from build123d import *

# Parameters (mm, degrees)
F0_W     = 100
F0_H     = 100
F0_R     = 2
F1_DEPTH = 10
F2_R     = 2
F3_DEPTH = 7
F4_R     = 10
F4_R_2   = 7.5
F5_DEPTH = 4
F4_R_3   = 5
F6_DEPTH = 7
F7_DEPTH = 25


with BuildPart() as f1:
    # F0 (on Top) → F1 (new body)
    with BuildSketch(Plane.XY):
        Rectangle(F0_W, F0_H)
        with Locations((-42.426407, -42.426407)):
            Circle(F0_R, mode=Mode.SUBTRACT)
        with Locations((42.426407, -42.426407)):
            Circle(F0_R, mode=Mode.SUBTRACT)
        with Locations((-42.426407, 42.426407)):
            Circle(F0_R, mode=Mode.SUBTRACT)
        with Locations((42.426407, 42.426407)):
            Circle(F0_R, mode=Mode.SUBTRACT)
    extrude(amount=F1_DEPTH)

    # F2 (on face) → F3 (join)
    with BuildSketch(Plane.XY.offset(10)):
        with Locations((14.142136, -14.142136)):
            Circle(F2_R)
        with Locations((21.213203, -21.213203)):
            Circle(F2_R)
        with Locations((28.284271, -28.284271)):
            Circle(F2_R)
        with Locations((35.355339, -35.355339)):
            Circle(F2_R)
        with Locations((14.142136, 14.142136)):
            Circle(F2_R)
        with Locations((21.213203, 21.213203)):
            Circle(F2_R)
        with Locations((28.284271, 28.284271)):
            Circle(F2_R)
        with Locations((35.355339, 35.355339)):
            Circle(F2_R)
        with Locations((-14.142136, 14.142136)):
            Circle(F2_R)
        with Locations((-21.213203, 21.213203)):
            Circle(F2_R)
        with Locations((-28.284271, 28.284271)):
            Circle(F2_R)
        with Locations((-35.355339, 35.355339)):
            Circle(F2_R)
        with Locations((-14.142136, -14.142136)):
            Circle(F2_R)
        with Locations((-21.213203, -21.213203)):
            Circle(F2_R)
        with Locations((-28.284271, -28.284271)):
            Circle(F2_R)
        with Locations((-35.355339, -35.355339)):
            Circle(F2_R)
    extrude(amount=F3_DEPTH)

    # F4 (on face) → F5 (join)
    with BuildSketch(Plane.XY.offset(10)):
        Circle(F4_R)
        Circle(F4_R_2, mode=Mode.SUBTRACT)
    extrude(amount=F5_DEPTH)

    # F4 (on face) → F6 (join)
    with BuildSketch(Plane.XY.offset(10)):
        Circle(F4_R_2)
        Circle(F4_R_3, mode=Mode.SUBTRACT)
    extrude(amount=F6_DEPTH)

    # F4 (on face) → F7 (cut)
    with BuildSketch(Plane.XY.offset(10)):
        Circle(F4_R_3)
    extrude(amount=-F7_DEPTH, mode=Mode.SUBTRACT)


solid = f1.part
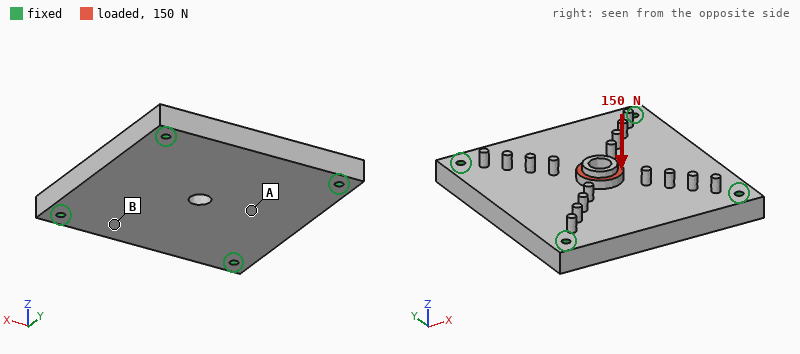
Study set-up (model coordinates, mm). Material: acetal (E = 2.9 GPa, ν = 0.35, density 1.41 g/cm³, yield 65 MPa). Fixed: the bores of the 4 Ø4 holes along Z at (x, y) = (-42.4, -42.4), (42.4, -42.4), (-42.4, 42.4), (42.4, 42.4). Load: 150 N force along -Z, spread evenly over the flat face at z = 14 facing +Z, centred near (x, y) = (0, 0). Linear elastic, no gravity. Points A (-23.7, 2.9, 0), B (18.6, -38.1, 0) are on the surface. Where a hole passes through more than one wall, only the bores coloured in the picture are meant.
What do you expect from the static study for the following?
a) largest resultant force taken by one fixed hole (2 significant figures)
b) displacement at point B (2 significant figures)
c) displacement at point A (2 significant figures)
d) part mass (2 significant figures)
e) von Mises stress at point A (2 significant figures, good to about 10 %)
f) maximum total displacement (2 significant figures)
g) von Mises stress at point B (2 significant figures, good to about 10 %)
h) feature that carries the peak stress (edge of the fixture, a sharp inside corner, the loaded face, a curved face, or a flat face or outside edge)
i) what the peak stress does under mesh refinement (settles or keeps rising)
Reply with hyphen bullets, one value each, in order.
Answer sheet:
- 38 N
- 23 µm
- 48 µm
- 140 g
- 0.90 MPa
- 68 µm
- 0.39 MPa
- edge of the fixture
- keeps rising
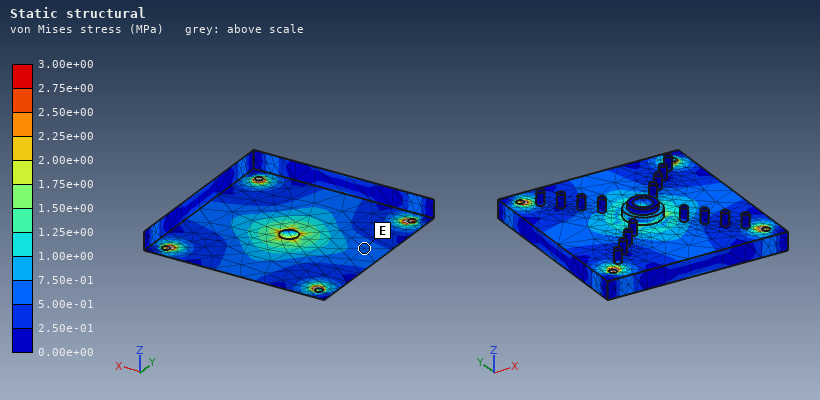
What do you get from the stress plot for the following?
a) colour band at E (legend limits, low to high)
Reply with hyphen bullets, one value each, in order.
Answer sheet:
- 5.00e-01 to 7.50e-01 MPa
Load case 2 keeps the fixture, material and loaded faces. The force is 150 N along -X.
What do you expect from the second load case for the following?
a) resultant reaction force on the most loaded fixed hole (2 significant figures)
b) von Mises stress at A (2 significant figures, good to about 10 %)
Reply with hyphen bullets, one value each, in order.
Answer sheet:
- 43 N
- 0.28 MPa
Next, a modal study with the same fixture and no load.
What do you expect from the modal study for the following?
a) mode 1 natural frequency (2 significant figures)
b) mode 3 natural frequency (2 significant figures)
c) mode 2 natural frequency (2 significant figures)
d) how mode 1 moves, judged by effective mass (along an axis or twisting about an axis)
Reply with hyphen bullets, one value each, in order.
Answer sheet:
- 1100 Hz
- 1900 Hz
- 1900 Hz
- along Z
